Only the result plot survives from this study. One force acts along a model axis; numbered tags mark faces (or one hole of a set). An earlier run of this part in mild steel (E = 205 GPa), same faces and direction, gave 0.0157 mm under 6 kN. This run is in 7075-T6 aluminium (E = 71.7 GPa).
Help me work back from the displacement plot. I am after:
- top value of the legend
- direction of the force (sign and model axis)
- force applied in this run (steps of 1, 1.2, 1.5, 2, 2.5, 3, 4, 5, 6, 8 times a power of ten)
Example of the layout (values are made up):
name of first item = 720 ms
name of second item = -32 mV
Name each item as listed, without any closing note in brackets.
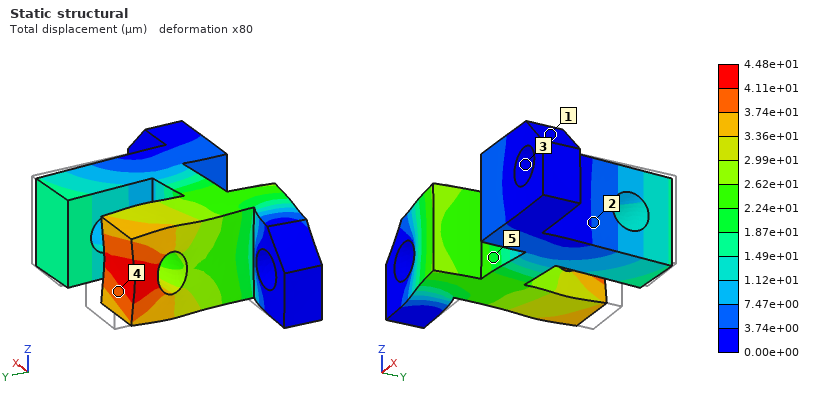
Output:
top value of the legend = 4.48e+01 µm
direction of the force = -Y
force applied in this run = 6 kN
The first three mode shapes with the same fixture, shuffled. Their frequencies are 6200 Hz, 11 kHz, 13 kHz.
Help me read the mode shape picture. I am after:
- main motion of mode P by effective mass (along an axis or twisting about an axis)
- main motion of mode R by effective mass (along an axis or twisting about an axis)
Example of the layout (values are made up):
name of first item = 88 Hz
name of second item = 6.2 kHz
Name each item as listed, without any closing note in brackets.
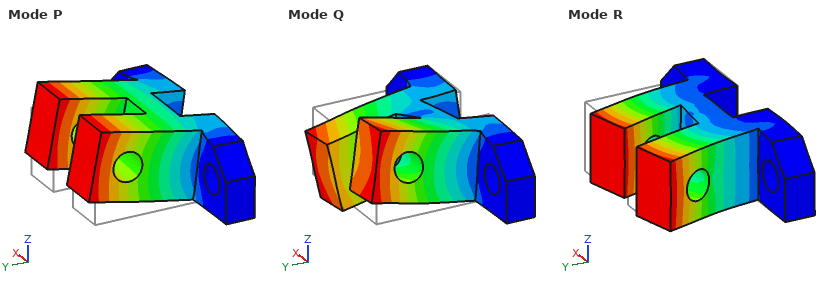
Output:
main motion of mode P by effective mass = along Z
main motion of mode R by effective mass = along X
